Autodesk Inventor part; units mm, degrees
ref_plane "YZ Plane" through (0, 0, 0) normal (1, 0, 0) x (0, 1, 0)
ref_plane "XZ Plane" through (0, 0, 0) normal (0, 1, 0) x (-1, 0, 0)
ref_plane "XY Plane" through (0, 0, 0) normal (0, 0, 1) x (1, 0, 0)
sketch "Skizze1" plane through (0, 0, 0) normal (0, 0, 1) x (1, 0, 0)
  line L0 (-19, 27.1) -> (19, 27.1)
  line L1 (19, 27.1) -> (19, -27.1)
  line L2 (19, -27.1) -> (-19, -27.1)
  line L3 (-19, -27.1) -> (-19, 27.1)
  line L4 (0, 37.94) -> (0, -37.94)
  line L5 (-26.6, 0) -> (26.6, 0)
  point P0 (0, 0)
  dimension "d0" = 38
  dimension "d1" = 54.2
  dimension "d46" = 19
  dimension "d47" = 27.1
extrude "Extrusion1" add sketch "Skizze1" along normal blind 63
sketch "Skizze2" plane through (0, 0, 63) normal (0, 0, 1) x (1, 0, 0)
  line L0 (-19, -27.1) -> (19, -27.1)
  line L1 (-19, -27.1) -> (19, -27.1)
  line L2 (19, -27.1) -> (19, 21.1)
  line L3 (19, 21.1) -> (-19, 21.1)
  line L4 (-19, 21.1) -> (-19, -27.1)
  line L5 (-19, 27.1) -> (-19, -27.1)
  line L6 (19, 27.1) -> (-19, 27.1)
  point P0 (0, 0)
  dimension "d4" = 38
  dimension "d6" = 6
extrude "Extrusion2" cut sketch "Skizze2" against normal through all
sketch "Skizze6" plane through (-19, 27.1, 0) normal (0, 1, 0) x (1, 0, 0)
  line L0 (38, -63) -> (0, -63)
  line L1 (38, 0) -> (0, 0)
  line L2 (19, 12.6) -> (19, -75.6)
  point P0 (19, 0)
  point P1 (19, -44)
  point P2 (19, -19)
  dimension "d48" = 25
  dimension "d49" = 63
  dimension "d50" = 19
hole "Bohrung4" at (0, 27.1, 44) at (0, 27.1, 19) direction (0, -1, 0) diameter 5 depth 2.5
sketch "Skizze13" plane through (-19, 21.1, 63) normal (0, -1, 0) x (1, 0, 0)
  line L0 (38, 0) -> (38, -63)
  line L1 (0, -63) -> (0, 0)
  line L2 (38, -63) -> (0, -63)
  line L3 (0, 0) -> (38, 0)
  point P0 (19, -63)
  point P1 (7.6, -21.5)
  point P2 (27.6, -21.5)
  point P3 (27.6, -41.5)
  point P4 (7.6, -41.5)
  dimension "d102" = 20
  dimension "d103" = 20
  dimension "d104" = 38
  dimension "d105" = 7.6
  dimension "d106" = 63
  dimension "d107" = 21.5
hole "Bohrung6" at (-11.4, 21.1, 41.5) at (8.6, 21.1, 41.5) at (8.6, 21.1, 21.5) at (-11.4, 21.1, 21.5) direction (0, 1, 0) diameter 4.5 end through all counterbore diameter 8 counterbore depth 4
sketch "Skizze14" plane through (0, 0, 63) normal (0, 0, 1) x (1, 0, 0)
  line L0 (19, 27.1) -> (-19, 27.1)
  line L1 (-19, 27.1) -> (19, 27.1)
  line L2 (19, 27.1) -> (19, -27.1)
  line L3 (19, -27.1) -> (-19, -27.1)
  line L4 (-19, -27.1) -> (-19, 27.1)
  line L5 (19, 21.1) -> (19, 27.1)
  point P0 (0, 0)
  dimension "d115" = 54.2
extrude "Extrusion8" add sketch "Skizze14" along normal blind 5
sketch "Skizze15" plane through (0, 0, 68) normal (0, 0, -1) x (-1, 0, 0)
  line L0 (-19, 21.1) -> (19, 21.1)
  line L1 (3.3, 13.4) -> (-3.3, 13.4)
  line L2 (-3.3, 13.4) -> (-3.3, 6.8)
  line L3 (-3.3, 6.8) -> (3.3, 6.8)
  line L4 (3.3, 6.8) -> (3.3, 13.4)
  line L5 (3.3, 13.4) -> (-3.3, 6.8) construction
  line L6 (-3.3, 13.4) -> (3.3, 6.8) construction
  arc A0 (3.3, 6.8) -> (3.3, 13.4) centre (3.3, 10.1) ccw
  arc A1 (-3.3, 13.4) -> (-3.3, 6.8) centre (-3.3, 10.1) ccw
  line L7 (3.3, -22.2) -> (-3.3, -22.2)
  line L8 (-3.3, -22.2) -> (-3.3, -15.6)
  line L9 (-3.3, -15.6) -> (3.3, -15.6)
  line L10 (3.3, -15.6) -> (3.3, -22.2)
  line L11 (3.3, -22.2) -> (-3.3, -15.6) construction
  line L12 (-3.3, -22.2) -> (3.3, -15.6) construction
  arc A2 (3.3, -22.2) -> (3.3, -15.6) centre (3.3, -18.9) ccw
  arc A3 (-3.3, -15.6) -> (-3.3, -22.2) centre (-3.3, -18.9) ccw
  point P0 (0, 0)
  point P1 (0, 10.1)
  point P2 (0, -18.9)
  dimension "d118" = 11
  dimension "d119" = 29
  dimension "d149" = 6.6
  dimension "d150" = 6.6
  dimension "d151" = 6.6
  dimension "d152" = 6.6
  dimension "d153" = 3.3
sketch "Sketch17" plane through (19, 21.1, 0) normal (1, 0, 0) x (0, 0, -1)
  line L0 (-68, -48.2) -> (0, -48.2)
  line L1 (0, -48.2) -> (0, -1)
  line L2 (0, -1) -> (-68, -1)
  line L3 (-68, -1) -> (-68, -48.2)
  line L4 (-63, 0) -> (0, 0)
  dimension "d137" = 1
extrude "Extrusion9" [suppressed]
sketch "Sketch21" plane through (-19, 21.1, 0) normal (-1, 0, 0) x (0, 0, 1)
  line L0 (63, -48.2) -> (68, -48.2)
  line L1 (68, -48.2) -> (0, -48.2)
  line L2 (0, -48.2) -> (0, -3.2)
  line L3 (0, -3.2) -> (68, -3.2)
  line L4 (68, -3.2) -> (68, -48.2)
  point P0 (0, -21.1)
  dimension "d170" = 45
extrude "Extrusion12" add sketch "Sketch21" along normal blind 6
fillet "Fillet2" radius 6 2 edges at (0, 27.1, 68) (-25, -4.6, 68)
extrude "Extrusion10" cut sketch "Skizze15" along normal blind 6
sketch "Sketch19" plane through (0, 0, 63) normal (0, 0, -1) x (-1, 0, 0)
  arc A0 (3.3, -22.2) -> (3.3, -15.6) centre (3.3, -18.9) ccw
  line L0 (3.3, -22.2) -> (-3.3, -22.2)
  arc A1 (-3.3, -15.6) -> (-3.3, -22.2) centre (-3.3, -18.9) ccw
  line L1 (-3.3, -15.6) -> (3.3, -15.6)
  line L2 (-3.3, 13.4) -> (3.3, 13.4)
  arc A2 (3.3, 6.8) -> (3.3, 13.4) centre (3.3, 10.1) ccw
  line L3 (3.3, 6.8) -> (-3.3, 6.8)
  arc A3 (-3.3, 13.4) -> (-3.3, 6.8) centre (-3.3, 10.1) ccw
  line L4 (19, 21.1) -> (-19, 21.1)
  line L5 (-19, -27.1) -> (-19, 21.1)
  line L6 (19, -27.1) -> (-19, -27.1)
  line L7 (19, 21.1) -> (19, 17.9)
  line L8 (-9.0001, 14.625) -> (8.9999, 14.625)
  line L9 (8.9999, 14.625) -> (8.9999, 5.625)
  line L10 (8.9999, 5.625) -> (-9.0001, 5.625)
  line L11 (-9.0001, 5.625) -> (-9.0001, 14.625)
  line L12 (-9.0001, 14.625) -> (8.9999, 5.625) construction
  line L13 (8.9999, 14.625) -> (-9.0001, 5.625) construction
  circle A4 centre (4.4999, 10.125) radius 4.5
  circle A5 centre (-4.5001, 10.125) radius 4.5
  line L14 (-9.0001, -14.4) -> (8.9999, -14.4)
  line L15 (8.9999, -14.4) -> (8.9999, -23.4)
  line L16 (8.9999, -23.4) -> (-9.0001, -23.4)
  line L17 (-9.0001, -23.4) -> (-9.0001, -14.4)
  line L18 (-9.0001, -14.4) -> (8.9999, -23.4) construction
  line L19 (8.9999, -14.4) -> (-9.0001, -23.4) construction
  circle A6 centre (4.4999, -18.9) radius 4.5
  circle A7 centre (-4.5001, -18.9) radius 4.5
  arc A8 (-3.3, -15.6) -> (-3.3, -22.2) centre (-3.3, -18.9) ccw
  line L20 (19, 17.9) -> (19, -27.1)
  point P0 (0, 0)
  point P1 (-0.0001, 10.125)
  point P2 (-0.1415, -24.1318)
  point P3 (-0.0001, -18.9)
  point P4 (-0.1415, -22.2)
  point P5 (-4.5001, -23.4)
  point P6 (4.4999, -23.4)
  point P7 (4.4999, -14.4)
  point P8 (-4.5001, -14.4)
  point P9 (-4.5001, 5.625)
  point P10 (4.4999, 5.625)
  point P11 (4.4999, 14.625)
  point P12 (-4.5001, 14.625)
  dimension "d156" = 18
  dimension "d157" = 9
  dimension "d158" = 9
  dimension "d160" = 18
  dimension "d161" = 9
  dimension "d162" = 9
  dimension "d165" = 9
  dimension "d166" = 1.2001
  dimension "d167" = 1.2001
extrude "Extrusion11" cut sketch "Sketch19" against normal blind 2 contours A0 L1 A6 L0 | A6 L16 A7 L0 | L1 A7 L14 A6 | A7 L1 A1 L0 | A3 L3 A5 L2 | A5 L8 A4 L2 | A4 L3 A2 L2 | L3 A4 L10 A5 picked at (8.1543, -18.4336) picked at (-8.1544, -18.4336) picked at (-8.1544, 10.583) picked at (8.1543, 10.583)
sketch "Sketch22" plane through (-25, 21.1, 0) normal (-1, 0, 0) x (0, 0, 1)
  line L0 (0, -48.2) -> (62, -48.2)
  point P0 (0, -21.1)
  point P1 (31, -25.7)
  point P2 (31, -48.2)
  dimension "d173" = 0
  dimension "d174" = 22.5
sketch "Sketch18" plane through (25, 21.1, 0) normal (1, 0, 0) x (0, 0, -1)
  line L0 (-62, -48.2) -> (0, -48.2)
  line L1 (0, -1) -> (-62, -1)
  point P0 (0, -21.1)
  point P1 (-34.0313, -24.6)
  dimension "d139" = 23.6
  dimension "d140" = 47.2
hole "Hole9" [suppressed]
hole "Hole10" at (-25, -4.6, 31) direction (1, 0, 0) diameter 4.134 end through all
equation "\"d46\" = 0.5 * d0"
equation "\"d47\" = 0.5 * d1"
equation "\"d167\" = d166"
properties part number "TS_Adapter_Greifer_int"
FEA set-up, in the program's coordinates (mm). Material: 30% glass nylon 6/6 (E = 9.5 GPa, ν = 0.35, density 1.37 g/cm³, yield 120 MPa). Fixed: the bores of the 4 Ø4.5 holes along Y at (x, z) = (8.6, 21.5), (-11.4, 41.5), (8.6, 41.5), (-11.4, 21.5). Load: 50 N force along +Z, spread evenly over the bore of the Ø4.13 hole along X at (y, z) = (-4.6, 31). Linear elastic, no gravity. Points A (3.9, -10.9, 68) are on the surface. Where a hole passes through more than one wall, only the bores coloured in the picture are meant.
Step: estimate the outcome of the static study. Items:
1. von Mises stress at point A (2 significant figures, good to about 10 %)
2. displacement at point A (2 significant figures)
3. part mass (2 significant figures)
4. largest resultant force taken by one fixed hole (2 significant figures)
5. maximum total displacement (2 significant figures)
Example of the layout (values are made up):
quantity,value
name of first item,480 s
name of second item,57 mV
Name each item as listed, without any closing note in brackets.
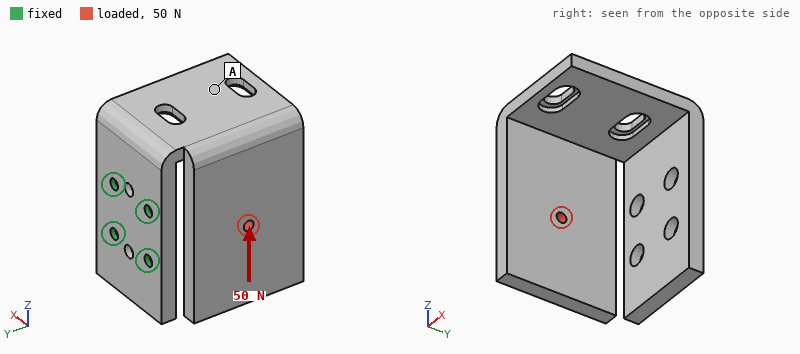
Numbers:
quantity,value
von Mises stress at point A,1.6 MPa
displacement at point A,0.37 mm
part mass,55 g
largest resultant force taken by one fixed hole,80 N
maximum total displacement,1.1 mm
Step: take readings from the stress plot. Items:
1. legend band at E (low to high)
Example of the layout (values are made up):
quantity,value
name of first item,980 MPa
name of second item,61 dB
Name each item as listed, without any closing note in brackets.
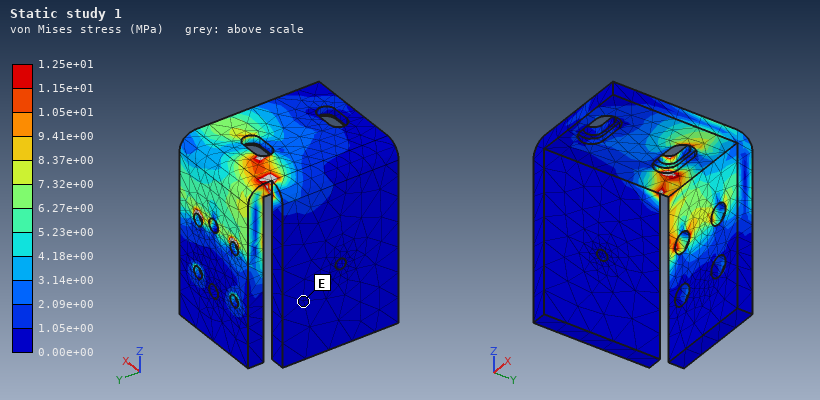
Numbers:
quantity,value
legend band at E,0.00e+00 to 1.05e+00 MPa
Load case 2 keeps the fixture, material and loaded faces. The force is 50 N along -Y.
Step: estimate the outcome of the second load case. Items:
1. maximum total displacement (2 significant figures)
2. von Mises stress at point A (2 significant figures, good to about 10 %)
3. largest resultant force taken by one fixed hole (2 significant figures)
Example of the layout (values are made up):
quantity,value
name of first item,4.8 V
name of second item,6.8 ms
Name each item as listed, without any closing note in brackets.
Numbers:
quantity,value
maximum total displacement,1.2 mm
von Mises stress at point A,1.7 MPa
largest resultant force taken by one fixed hole,67 N
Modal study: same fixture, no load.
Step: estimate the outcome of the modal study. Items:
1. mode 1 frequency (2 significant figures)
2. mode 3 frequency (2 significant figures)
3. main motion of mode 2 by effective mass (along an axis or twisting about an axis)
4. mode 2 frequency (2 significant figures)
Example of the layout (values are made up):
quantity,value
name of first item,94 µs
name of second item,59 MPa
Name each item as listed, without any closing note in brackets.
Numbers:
quantity,value
mode 1 frequency,210 Hz
mode 3 frequency,640 Hz
main motion of mode 2 by effective mass,along X
mode 2 frequency,290 Hz
